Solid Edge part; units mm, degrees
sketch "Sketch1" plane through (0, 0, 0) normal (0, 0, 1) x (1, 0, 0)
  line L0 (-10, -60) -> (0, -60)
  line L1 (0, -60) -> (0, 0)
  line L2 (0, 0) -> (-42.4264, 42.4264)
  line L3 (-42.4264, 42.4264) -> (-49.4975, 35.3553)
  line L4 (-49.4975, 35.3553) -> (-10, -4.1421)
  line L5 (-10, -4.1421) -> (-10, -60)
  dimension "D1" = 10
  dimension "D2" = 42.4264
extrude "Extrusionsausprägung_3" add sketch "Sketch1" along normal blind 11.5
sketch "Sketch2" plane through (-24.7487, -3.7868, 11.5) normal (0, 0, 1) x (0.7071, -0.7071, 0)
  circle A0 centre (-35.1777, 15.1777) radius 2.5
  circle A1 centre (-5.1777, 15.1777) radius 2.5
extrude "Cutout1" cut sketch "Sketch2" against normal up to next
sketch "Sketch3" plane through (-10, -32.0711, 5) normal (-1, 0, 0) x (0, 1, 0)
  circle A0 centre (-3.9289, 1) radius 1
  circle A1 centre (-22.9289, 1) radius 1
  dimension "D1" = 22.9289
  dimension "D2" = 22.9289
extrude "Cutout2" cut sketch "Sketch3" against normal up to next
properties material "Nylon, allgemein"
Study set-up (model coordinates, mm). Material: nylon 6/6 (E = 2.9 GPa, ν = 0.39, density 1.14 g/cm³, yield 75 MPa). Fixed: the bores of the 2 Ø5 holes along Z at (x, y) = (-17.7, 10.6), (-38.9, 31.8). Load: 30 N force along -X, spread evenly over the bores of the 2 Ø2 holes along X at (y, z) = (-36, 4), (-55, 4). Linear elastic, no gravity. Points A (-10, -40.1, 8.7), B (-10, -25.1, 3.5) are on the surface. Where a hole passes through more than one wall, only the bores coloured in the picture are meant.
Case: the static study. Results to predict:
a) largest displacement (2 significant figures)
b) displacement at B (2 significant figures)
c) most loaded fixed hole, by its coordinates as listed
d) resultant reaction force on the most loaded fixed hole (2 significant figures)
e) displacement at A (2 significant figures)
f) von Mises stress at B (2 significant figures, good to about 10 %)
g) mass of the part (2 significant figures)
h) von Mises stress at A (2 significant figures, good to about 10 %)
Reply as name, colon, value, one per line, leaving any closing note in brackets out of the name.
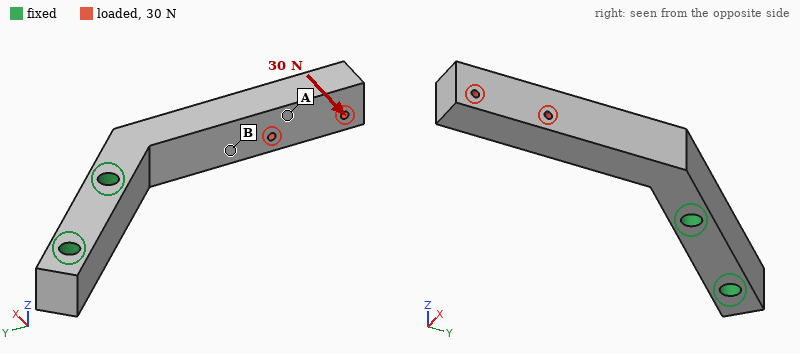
largest displacement: 1.1 mm
displacement at B: 0.40 mm
most loaded fixed hole, by its coordinates as listed: (-17.7, 10.6)
resultant reaction force on the most loaded fixed hole: 37 N
displacement at A: 0.68 mm
von Mises stress at B: 3.2 MPa
mass of the part: 15 g
von Mises stress at A: 1.2 MPa
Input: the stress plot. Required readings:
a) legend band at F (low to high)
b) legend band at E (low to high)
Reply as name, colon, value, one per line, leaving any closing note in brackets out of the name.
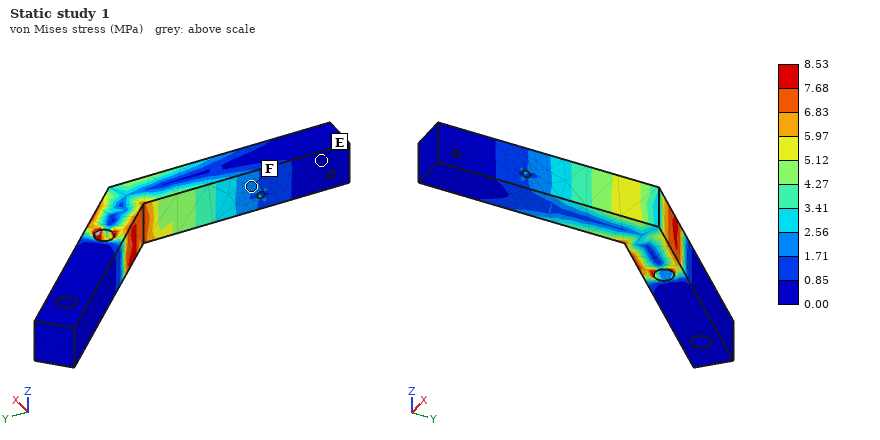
legend band at F: 1.71 to 2.56 MPa
legend band at E: 0.00 to 0.85 MPa
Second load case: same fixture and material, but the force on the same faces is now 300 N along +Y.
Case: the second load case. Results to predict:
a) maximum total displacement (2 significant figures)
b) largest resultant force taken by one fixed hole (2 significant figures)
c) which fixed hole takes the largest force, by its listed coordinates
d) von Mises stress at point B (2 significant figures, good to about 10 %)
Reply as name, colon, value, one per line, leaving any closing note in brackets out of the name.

maximum total displacement: 1.1 mm
largest resultant force taken by one fixed hole: 310 N
which fixed hole takes the largest force, by its listed coordinates: (-17.7, 10.6)
von Mises stress at point B: 3.5 MPa
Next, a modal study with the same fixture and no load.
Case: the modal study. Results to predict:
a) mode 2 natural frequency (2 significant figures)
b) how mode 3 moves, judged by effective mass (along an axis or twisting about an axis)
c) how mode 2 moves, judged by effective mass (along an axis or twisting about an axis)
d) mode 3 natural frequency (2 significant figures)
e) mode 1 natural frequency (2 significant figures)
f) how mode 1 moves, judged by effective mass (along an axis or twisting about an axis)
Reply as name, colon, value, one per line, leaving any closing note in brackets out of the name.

mode 2 natural frequency: 510 Hz
how mode 3 moves, judged by effective mass: along Y
how mode 2 moves, judged by effective mass: along Z
mode 3 natural frequency: 2400 Hz
mode 1 natural frequency: 460 Hz
how mode 1 moves, judged by effective mass: along X
